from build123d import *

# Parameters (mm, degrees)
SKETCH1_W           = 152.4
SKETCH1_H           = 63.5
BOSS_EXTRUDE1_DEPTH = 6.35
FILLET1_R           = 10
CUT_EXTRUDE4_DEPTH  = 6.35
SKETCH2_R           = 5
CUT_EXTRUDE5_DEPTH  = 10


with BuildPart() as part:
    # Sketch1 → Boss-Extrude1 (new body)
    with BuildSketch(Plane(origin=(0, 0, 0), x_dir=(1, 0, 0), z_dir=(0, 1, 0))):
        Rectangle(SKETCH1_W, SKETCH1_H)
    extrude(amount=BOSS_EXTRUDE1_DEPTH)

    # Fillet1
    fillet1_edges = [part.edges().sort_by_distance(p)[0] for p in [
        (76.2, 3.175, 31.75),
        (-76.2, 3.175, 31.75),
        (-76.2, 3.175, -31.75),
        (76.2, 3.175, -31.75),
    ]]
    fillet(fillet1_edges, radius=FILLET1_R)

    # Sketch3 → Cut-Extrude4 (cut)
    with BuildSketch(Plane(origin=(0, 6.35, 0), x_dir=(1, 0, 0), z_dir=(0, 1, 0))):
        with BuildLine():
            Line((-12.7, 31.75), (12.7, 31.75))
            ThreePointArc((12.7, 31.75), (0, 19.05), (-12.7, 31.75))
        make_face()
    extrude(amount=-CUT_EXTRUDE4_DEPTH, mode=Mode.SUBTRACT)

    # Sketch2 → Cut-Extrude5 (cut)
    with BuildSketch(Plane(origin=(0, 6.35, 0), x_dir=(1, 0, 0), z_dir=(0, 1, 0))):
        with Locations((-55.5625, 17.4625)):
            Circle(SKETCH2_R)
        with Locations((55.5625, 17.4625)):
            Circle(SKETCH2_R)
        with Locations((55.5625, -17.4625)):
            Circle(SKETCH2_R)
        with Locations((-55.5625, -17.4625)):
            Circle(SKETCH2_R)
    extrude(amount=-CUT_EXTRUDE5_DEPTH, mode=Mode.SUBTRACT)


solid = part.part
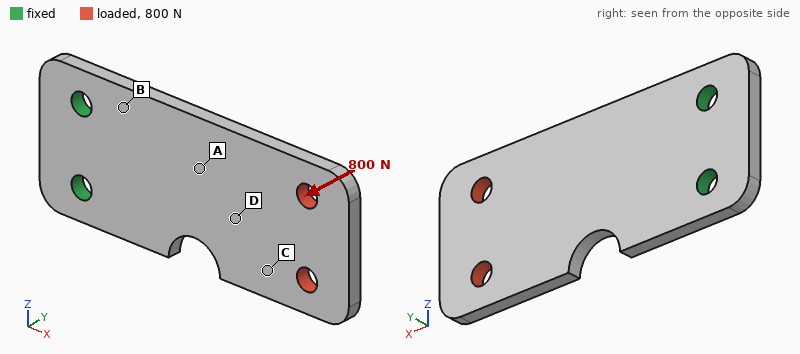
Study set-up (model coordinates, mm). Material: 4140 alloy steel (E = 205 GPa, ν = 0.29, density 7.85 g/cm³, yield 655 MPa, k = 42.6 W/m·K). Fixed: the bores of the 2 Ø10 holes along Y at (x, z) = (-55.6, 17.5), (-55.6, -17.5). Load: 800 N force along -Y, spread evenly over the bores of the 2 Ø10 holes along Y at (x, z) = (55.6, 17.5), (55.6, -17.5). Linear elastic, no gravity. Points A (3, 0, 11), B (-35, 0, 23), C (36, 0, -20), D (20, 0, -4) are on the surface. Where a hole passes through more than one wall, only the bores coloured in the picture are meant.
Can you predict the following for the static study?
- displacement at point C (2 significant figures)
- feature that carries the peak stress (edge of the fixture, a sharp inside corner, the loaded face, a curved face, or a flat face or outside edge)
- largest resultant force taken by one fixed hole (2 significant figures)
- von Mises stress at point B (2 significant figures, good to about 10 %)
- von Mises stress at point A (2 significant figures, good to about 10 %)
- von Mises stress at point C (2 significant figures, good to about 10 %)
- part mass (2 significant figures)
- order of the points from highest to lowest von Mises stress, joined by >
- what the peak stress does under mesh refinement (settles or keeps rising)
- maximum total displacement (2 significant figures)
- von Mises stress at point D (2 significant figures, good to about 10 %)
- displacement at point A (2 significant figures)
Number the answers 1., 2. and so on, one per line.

1. 0.94 mm
2. edge of the fixture
3. 400 N
4. 170 MPa
5. 110 MPa
6. 34 MPa
7. 450 g
8. B > A > D > C
9. keeps rising
10. 1.7 mm
11. 71 MPa
12. 0.41 mm
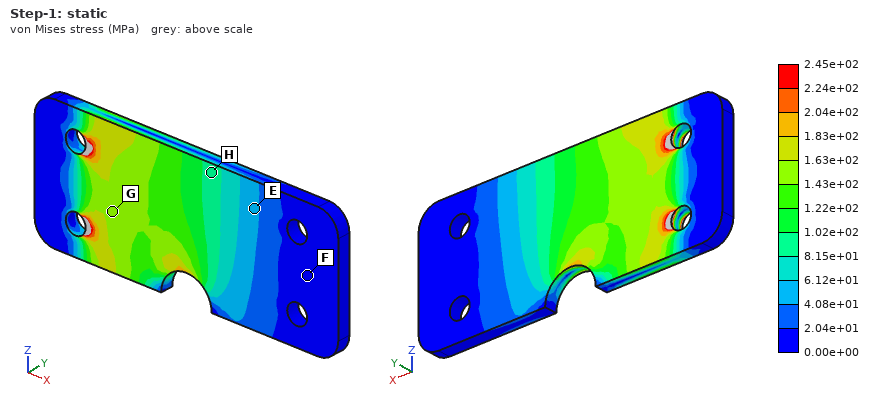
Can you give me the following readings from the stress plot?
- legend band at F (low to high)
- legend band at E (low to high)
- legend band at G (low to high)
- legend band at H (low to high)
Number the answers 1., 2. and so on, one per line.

1. 0.00e+00 to 2.04e+01 MPa
2. 4.08e+01 to 6.12e+01 MPa
3. 1.43e+02 to 1.63e+02 MPa
4. 8.15e+01 to 1.02e+02 MPa
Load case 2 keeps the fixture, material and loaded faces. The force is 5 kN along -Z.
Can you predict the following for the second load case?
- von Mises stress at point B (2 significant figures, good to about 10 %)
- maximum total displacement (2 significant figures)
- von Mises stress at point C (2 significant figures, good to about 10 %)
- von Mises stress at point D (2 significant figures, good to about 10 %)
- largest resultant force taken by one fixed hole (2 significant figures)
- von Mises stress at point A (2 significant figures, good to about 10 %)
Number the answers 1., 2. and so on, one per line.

1. 84 MPa
2. 0.17 mm
3. 17 MPa
4. 44 MPa
5. 14 kN
6. 42 MPa
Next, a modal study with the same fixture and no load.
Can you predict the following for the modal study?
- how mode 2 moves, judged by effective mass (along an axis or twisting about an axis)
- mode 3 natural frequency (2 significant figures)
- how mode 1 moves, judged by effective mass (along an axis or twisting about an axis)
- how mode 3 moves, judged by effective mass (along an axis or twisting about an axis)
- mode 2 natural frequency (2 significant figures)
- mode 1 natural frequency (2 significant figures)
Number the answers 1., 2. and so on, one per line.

1. twisting about X
2. 2000 Hz
3. along Y
4. along Y
5. 1300 Hz
6. 320 Hz
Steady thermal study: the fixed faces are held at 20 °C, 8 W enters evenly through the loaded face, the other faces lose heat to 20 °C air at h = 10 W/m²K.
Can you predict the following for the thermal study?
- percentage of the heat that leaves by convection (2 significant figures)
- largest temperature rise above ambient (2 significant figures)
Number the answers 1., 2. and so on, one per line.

1. 44 %
2. 38 K
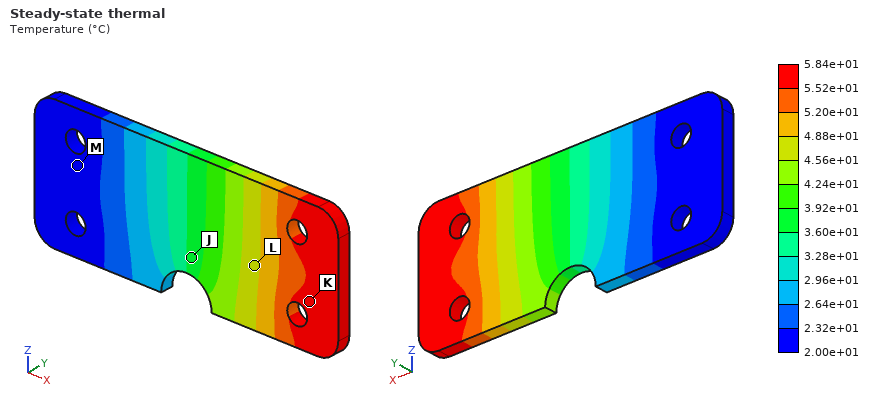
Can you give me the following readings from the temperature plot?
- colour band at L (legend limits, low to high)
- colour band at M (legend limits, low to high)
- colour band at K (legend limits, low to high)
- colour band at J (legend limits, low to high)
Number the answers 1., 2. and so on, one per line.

1. 4.56e+01 to 4.88e+01 °C
2. 2.00e+01 to 2.32e+01 °C
3. 5.52e+01 to 5.84e+01 °C
4. 3.60e+01 to 3.92e+01 °C
